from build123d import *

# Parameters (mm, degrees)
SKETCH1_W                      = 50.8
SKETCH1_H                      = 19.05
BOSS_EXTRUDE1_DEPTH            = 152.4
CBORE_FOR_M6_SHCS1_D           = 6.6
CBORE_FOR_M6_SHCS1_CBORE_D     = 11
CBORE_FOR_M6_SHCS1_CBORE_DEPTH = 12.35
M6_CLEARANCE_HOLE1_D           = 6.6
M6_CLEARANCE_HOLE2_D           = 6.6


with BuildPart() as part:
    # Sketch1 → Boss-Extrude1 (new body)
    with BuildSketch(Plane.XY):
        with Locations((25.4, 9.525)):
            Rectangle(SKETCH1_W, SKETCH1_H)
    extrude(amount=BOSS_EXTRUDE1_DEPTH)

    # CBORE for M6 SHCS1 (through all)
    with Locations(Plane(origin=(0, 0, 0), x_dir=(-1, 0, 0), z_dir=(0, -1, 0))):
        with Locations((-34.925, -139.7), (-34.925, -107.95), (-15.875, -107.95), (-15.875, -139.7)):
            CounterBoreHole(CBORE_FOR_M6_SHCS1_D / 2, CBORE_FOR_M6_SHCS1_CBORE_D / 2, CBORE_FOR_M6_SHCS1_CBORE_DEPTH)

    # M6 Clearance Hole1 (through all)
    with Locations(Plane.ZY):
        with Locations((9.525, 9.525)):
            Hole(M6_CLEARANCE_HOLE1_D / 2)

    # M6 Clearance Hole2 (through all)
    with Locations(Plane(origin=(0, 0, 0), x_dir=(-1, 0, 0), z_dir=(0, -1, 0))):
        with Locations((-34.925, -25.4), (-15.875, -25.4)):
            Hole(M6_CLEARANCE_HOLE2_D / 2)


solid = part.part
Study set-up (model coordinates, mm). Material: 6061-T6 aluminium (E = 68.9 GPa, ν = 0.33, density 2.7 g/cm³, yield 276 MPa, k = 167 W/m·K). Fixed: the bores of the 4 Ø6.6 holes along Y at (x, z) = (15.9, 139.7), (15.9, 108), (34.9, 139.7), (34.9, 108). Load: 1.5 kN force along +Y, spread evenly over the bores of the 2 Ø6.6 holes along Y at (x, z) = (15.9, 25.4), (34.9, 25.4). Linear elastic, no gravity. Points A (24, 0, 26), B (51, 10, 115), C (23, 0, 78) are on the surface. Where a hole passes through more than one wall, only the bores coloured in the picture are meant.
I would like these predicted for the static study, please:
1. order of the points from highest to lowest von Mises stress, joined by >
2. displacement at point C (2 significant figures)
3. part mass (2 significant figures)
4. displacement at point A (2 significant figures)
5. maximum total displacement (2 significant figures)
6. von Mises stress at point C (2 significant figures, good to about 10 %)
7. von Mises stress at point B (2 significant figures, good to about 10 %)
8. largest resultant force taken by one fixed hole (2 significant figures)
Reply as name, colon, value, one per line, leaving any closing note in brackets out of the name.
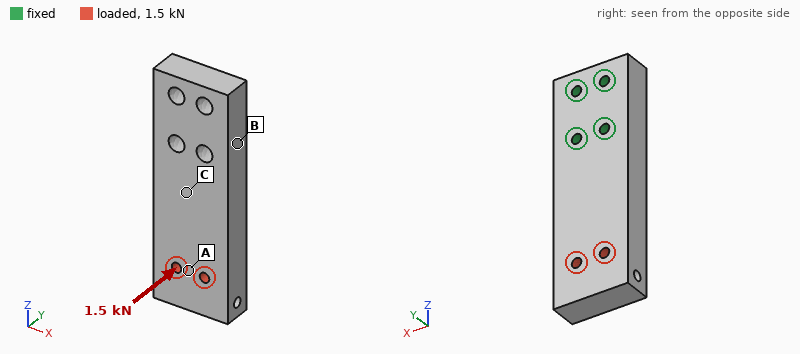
order of the points from highest to lowest von Mises stress, joined by >: C > B > A
displacement at point C: 0.058 mm
part mass: 370 g
displacement at point A: 0.21 mm
maximum total displacement: 0.29 mm
von Mises stress at point C: 23 MPa
von Mises stress at point B: 14 MPa
largest resultant force taken by one fixed hole: 2.9 kN
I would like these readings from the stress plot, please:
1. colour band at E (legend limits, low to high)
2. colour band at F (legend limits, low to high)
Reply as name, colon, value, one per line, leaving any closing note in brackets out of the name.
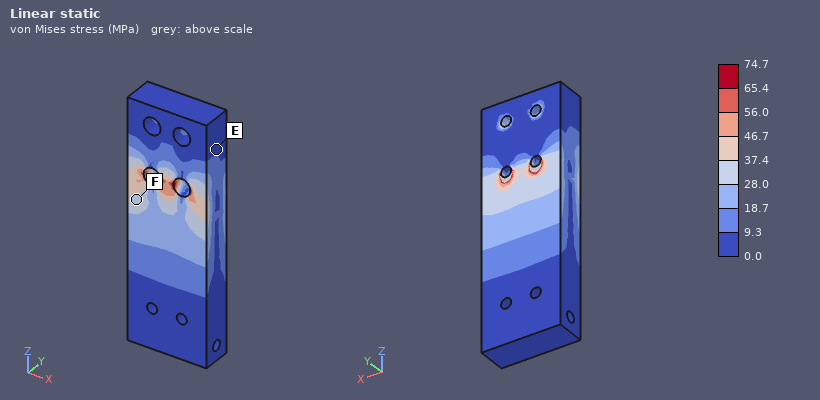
colour band at E: 0.0 to 9.3 MPa
colour band at F: 28.0 to 37.4 MPa
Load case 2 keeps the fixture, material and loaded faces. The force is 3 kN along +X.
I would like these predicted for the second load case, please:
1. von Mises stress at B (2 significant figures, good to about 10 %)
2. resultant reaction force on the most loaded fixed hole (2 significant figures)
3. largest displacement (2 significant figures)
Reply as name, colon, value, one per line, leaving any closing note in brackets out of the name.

von Mises stress at B: 23 MPa
resultant reaction force on the most loaded fixed hole: 5.7 kN
largest displacement: 0.11 mm
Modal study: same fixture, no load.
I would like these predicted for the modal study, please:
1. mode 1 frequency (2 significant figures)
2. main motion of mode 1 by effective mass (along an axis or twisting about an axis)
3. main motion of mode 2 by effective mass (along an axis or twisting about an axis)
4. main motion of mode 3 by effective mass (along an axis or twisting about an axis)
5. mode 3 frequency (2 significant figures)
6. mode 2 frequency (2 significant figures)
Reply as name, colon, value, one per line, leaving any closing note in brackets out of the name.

mode 1 frequency: 1100 Hz
main motion of mode 1 by effective mass: along Y
main motion of mode 2 by effective mass: along X
main motion of mode 3 by effective mass: twisting about Z
mode 3 frequency: 4200 Hz
mode 2 frequency: 2500 Hz
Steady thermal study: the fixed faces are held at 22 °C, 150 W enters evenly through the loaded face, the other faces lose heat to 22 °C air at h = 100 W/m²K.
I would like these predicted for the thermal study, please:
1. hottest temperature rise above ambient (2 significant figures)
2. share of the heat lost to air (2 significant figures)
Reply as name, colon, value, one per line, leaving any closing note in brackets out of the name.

hottest temperature rise above ambient: 59 K
share of the heat lost to air: 43 %
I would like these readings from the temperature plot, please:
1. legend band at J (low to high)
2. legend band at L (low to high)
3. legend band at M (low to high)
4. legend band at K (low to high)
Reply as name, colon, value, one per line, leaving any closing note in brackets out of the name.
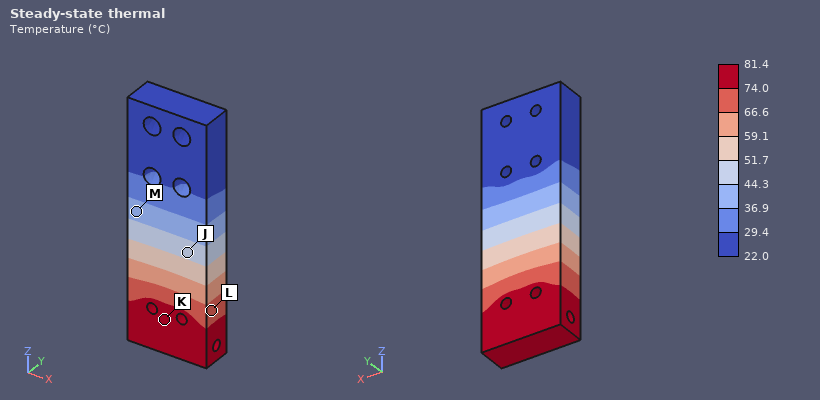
legend band at J: 44.3 to 51.7 °C
legend band at L: 66.6 to 74.0 °C
legend band at M: 36.9 to 44.3 °C
legend band at K: 74.0 to 81.4 °C
